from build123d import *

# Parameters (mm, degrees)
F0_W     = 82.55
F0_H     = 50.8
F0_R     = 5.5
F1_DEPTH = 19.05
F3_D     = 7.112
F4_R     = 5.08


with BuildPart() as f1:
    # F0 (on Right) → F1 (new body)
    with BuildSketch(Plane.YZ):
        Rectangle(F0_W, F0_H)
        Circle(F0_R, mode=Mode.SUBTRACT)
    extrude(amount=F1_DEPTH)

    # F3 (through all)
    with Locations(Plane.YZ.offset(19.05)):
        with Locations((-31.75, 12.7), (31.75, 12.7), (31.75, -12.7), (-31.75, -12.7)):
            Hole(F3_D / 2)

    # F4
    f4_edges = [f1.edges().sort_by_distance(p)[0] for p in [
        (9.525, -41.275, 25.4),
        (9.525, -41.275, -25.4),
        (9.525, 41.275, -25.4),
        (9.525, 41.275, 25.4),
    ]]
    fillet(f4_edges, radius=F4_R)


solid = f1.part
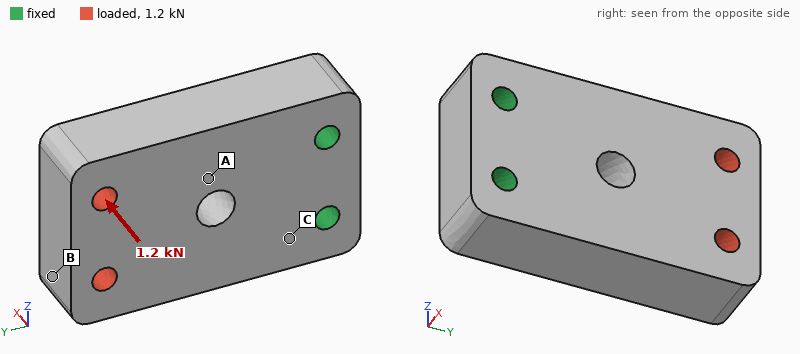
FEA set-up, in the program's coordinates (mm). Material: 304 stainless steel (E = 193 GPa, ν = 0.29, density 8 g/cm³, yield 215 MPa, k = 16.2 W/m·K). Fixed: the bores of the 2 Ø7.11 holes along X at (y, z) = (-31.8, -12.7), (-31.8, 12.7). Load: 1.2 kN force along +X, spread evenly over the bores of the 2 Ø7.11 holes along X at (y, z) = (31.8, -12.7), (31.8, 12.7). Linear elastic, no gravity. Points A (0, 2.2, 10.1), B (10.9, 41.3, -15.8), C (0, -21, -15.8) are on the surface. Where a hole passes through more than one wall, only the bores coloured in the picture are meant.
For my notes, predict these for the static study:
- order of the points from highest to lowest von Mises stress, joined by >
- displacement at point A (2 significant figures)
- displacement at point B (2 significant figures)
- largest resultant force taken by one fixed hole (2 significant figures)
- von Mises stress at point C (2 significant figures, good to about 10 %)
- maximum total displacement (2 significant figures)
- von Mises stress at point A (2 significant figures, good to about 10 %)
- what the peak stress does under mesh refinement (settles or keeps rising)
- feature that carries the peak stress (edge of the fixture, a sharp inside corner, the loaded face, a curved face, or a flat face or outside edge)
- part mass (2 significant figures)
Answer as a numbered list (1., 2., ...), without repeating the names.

1. C > A > B
2. 8.4 µm
3. 25 µm
4. 600 N
5. 23 MPa
6. 26 µm
7. 13 MPa
8. keeps rising
9. edge of the fixture
10. 600 g
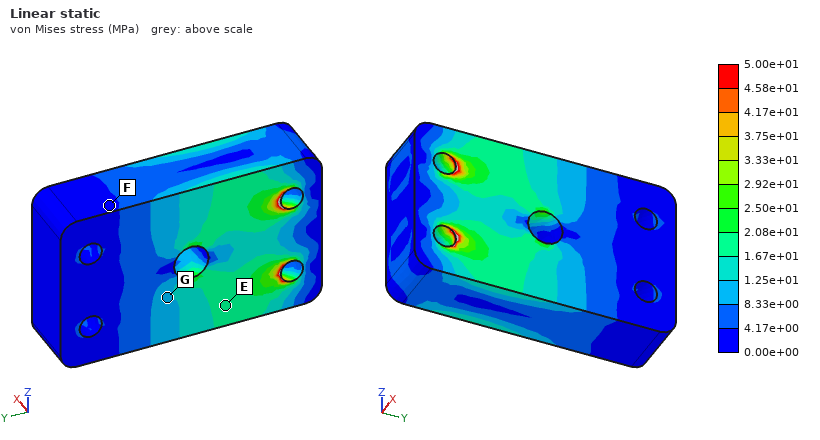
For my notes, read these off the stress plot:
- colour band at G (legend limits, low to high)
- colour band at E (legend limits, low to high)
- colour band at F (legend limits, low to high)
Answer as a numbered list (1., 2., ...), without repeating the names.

1. 8.33e+00 to 1.25e+01 MPa
2. 1.67e+01 to 2.08e+01 MPa
3. 0.00e+00 to 4.17e+00 MPa
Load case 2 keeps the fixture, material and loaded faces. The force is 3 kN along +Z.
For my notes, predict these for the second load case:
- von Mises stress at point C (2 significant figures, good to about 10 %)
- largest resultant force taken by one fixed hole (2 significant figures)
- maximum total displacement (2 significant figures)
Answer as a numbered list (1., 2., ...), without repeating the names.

1. 15 MPa
2. 6.3 kN
3. 15 µm
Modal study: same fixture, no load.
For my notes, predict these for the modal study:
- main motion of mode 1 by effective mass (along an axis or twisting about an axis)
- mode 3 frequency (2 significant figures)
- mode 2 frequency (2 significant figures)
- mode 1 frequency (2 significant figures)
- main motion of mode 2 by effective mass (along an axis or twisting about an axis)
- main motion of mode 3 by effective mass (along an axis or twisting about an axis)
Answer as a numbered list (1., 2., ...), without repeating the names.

1. along X
2. 7000 Hz
3. 5200 Hz
4. 2700 Hz
5. along Z
6. twisting about Y
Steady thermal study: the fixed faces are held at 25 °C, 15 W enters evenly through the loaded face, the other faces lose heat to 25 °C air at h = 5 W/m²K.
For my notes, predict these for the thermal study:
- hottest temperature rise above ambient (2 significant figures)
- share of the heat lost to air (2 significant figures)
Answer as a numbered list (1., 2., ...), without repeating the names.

1. 63 K
2. 13 %
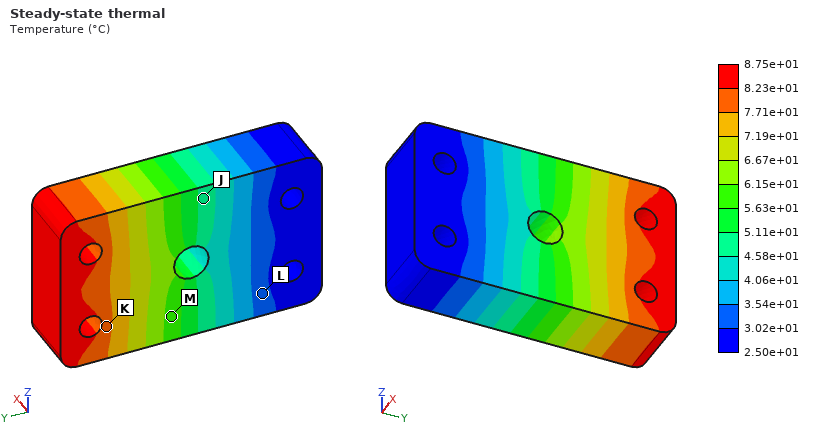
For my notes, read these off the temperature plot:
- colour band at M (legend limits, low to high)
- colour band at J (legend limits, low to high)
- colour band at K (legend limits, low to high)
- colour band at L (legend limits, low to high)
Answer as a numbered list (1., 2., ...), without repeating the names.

1. 5.63e+01 to 6.15e+01 °C
2. 4.58e+01 to 5.11e+01 °C
3. 7.71e+01 to 8.23e+01 °C
4. 3.02e+01 to 3.54e+01 °C
